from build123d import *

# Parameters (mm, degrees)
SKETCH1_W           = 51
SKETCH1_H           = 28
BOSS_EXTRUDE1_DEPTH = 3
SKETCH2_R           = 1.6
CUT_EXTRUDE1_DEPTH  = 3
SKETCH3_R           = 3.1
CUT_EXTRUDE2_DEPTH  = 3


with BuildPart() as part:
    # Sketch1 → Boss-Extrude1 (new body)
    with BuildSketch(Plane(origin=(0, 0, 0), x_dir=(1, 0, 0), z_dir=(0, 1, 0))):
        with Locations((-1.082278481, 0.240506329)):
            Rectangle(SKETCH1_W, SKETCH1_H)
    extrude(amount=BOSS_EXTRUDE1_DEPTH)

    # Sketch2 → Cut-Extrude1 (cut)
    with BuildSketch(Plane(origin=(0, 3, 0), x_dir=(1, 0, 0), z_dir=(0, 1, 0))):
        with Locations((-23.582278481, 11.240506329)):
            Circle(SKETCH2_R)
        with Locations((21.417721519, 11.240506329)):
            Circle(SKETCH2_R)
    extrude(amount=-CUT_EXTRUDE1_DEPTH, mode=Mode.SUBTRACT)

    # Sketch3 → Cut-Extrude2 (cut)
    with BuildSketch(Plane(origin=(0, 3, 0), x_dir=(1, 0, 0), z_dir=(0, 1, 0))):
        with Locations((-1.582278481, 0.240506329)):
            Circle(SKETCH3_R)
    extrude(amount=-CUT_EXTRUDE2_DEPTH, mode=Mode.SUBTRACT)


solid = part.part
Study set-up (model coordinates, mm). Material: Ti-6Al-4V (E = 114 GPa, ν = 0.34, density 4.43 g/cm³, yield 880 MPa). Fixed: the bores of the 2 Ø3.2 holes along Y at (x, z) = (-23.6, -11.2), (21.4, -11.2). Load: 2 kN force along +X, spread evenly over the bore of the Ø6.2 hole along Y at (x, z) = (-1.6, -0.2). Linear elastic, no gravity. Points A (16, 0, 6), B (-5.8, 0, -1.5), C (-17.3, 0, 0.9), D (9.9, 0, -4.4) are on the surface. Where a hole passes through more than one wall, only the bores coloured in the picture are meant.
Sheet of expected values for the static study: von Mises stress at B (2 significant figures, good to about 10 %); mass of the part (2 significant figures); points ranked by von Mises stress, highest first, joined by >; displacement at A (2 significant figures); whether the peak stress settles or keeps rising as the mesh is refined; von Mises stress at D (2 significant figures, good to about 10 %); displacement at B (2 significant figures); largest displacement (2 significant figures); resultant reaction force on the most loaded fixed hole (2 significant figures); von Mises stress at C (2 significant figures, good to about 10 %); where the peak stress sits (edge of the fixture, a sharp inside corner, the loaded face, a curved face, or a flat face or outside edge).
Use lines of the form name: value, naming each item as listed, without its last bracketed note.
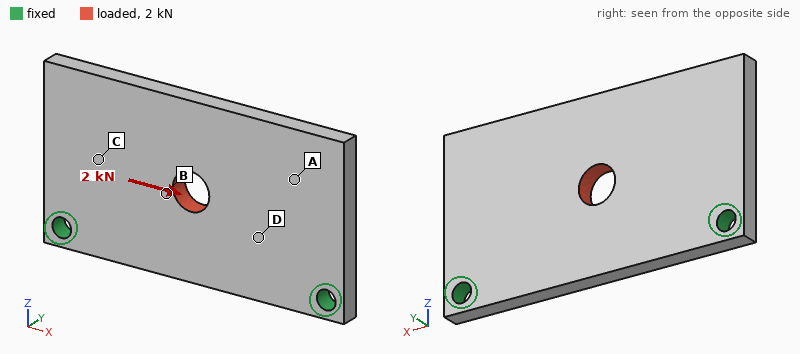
von Mises stress at B: 36 MPa
mass of the part: 18 g
points ranked by von Mises stress, highest first, joined by >: B > D > C > A
displacement at A: 6.3 µm
whether the peak stress settles or keeps rising as the mesh is refined: keeps rising
von Mises stress at D: 28 MPa
displacement at B: 6.6 µm
largest displacement: 8.7 µm
resultant reaction force on the most loaded fixed hole: 1.1 kN
von Mises stress at C: 13 MPa
where the peak stress sits: edge of the fixture
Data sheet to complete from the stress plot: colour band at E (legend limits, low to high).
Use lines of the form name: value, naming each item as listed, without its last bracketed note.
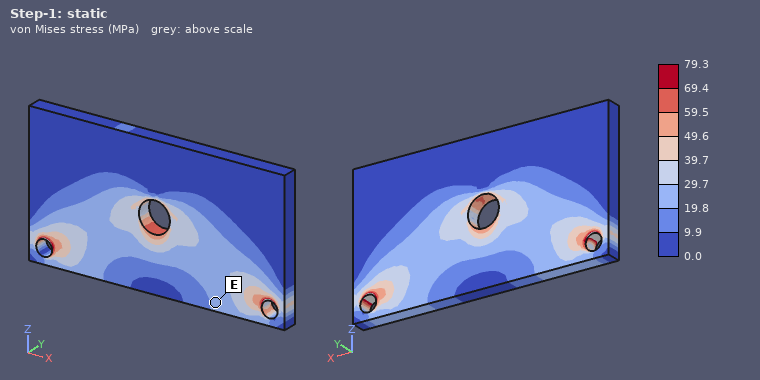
colour band at E: 19.8 to 29.7 MPa
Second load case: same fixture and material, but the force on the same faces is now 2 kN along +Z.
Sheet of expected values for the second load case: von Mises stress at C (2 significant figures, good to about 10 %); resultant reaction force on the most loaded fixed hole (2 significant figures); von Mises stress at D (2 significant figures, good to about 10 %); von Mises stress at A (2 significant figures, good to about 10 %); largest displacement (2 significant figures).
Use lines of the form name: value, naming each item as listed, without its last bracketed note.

von Mises stress at C: 26 MPa
resultant reaction force on the most loaded fixed hole: 1.2 kN
von Mises stress at D: 28 MPa
von Mises stress at A: 17 MPa
largest displacement: 13 µm
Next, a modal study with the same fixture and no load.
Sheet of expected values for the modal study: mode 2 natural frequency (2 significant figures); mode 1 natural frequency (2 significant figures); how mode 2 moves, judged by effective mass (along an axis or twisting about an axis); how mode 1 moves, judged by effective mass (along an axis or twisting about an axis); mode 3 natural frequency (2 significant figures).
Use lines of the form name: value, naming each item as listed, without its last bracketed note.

mode 2 natural frequency: 5700 Hz
mode 1 natural frequency: 2700 Hz
how mode 2 moves, judged by effective mass: twisting about Z
how mode 1 moves, judged by effective mass: along Y
mode 3 natural frequency: 7600 Hz
